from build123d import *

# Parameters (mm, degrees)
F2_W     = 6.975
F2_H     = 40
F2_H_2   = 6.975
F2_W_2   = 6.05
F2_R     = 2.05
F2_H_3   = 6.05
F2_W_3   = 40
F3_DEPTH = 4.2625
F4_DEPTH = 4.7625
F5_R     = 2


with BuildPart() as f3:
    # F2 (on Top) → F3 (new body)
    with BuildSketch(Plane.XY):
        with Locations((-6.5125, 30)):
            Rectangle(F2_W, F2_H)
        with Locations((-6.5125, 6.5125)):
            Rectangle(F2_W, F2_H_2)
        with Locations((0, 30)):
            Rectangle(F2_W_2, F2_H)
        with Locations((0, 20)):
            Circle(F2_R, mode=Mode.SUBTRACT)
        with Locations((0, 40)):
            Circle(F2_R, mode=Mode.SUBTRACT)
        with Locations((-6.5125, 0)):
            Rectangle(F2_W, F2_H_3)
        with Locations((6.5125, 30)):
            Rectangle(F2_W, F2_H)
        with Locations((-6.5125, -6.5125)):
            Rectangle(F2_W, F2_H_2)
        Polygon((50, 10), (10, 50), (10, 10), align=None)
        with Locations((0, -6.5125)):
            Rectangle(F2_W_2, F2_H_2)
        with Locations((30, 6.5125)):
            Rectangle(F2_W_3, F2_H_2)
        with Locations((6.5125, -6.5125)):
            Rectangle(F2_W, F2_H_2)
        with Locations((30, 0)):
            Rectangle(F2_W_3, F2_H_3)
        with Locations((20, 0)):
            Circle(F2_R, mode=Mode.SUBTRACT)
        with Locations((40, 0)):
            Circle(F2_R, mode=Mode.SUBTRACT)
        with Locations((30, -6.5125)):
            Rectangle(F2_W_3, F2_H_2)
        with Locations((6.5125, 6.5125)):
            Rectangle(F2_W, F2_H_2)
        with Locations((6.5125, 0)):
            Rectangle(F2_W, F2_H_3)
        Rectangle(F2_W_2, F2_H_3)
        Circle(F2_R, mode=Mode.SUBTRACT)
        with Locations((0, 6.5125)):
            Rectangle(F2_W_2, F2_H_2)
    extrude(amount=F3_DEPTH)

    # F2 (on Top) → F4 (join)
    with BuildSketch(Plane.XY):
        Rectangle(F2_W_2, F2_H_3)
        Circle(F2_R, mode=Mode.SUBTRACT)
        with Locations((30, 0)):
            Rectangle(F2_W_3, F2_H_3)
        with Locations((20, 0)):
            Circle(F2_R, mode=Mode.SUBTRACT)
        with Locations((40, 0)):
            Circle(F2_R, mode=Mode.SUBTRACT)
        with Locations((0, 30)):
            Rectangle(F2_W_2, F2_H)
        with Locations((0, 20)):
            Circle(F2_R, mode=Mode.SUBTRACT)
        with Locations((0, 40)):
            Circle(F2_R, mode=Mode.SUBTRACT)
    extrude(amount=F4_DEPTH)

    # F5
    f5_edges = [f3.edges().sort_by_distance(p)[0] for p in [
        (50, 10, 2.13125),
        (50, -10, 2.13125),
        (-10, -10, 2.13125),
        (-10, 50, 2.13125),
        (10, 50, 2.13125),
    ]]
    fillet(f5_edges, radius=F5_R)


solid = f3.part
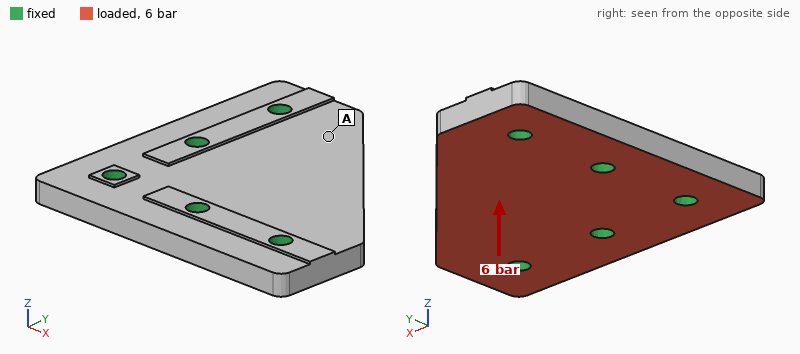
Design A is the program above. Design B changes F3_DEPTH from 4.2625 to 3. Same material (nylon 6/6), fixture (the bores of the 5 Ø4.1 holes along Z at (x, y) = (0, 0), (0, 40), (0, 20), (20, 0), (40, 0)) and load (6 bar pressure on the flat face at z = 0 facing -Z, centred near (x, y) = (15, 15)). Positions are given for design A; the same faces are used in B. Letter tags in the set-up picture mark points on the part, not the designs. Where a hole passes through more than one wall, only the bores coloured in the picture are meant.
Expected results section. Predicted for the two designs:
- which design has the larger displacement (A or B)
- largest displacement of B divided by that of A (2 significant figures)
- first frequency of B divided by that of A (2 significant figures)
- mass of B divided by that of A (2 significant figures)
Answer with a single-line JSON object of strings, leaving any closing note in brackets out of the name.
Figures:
{"which design has the larger displacement": "B", "largest displacement of B divided by that of A": "2.4", "first frequency of B divided by that of A": "0.77", "mass of B divided by that of A": "0.76"}
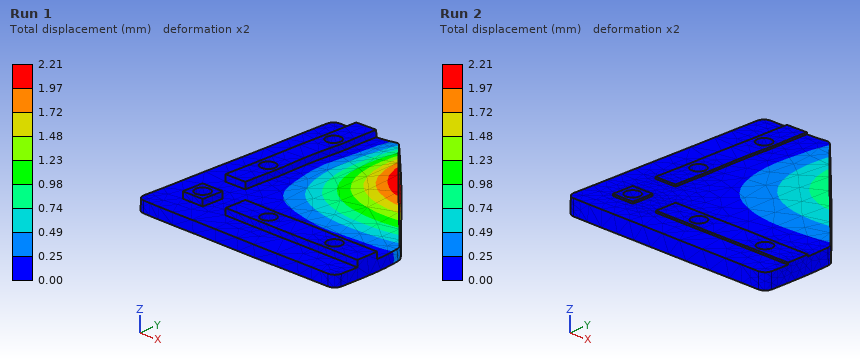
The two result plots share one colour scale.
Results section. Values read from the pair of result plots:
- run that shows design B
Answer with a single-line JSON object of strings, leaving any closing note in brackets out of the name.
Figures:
{"run that shows design B": "Run 1"}
